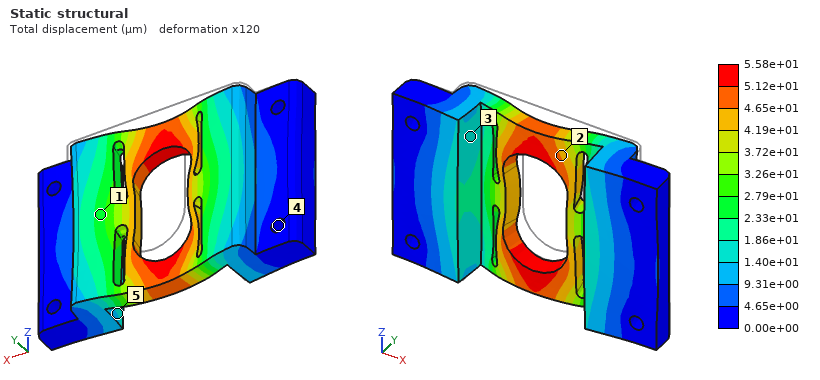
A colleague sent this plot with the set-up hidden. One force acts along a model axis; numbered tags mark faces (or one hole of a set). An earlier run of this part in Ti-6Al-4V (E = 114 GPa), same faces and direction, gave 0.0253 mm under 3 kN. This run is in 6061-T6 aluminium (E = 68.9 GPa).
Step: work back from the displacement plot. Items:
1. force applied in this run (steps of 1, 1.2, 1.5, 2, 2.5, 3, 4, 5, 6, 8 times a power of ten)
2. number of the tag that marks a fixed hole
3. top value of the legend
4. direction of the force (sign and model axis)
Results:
4 kN
4
5.58e+01 µm
-Y
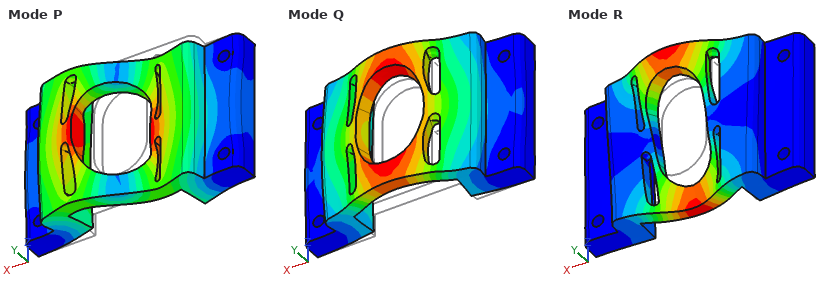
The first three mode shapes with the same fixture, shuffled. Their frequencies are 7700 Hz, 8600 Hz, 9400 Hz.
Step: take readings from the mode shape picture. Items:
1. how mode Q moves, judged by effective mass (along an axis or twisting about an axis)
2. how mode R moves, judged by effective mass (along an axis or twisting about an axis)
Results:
along Y
twisting about X
